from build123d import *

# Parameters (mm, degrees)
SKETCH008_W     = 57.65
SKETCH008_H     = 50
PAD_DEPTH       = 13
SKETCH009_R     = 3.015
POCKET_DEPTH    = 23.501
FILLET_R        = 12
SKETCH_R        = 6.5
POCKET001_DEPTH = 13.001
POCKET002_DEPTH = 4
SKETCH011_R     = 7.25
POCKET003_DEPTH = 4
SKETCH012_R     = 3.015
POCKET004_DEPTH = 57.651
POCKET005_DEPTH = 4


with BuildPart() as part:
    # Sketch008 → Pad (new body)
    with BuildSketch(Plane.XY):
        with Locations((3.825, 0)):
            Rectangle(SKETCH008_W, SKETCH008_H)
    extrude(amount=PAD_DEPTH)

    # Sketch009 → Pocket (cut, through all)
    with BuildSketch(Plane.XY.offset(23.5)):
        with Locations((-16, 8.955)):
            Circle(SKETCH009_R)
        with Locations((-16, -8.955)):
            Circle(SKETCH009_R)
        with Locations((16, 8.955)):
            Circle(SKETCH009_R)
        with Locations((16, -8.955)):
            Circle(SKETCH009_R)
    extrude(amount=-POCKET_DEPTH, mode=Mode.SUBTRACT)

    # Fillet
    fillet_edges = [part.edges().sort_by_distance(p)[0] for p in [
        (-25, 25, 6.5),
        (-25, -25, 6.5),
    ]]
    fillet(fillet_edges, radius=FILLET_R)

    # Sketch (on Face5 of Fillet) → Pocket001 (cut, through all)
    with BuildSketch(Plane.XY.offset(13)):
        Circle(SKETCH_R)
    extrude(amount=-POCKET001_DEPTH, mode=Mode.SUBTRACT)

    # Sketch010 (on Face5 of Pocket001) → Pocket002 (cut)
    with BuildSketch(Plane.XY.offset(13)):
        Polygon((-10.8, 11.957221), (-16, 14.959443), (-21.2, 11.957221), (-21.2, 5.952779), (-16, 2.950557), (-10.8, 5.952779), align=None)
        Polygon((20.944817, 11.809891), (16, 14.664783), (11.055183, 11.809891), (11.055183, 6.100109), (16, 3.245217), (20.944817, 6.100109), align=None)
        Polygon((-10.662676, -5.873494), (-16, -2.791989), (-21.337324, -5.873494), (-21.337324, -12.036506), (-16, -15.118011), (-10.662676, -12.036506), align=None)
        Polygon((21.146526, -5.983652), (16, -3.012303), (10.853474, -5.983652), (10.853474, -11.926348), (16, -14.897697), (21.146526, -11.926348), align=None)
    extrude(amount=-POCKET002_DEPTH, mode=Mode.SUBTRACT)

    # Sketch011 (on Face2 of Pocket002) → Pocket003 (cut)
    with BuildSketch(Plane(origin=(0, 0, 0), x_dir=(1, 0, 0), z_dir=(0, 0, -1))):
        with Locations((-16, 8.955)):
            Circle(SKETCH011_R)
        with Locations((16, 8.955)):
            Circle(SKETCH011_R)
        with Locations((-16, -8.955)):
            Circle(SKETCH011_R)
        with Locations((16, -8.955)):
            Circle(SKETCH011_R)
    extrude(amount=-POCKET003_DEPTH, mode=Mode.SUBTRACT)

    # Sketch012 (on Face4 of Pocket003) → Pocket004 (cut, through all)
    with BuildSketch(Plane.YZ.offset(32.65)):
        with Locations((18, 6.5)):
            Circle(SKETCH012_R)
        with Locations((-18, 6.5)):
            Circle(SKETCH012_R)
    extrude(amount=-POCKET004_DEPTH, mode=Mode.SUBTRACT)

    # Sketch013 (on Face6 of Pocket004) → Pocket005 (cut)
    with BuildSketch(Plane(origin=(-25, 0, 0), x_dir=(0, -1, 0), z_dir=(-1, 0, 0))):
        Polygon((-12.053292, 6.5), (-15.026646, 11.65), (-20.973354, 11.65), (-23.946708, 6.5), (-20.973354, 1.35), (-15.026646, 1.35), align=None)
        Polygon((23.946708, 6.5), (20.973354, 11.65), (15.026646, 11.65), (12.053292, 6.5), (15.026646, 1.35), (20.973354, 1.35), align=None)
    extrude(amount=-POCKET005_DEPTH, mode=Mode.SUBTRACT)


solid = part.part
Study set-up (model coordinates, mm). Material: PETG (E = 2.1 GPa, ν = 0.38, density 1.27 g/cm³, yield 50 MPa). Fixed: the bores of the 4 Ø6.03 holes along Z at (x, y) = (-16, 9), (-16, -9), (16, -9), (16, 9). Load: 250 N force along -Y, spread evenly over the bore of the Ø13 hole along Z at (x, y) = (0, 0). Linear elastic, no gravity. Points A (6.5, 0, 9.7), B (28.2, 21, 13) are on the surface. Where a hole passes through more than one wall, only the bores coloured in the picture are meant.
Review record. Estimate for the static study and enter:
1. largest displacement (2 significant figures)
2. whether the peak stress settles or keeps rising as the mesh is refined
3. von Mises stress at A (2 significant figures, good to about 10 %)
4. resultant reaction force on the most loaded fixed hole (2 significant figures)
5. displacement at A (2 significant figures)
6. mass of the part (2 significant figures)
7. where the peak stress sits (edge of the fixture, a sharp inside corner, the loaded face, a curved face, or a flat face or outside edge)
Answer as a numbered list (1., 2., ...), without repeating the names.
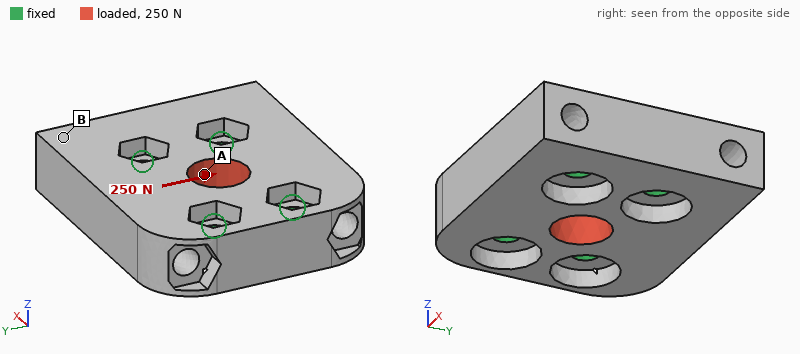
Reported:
1. 7.6 µm
2. keeps rising
3. 0.88 MPa
4. 65 N
5. 5.6 µm
6. 34 g
7. edge of the fixture
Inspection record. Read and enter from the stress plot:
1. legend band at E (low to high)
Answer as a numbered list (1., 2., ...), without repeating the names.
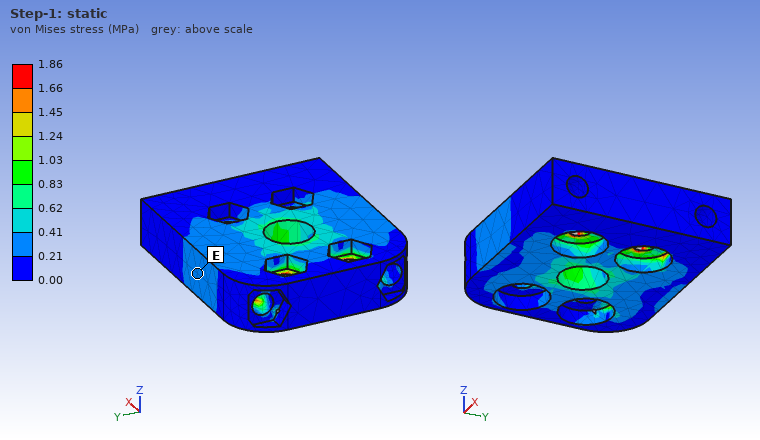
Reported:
1. 0.21 to 0.41 MPa
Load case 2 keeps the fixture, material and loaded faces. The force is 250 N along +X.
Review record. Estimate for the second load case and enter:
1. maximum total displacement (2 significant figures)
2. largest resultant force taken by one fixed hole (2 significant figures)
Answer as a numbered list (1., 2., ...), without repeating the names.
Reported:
1. 5.0 µm
2. 65 N
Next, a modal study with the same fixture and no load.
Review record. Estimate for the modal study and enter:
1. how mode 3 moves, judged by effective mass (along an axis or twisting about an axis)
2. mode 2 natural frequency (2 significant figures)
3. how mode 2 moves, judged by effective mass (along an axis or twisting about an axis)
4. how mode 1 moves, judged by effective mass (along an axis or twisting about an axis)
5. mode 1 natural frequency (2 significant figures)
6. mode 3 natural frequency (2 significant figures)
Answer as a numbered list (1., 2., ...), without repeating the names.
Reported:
1. along Z
2. 3700 Hz
3. along Z
4. twisting about X
5. 3400 Hz
6. 4000 Hz
